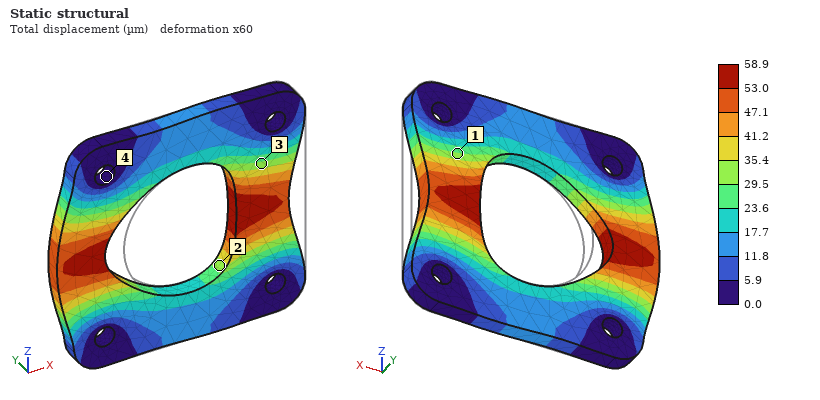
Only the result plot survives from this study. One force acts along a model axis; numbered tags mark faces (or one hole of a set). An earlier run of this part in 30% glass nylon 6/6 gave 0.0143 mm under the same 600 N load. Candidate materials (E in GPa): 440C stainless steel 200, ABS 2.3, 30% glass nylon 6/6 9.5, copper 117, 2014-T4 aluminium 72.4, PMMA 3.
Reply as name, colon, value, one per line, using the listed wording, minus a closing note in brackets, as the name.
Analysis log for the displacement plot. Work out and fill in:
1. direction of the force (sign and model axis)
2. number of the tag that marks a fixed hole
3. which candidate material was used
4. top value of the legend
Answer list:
direction of the force: -X
number of the tag that marks a fixed hole: 4
which candidate material was used: ABS
top value of the legend: 58.9 µm
